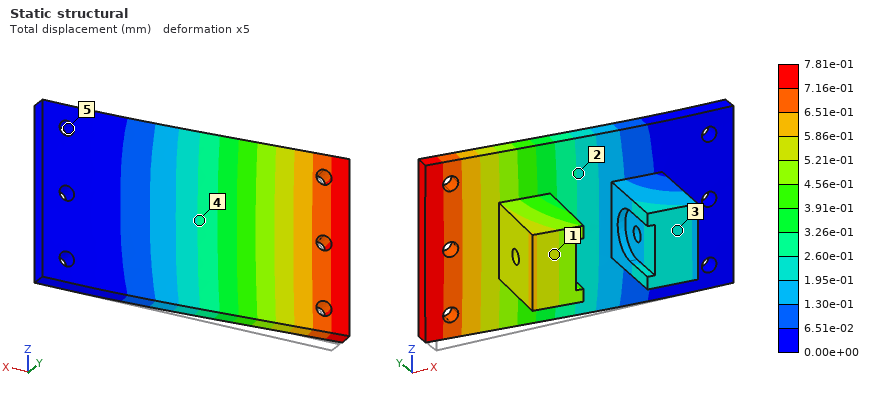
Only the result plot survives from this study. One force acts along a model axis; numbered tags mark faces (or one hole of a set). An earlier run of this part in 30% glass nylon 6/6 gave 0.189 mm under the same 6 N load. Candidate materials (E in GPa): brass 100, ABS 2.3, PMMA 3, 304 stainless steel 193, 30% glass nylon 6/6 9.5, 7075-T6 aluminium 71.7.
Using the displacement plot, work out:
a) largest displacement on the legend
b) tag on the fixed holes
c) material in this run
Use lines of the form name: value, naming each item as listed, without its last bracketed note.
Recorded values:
largest displacement on the legend: 7.81e-01 mm
tag on the fixed holes: 5
material in this run: ABS
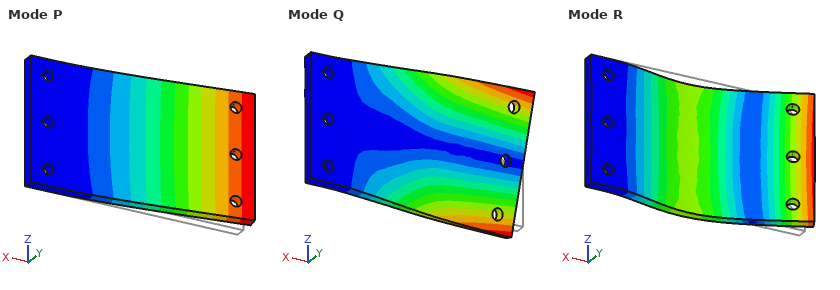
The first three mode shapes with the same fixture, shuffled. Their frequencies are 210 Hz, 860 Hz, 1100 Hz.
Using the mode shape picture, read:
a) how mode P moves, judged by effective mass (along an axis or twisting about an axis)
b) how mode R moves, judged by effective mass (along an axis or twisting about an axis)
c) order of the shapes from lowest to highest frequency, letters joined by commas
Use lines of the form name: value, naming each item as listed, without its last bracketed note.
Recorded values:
how mode P moves, judged by effective mass: along Y
how mode R moves, judged by effective mass: along Y
order of the shapes from lowest to highest frequency, letters joined by commas: P, Q, R
